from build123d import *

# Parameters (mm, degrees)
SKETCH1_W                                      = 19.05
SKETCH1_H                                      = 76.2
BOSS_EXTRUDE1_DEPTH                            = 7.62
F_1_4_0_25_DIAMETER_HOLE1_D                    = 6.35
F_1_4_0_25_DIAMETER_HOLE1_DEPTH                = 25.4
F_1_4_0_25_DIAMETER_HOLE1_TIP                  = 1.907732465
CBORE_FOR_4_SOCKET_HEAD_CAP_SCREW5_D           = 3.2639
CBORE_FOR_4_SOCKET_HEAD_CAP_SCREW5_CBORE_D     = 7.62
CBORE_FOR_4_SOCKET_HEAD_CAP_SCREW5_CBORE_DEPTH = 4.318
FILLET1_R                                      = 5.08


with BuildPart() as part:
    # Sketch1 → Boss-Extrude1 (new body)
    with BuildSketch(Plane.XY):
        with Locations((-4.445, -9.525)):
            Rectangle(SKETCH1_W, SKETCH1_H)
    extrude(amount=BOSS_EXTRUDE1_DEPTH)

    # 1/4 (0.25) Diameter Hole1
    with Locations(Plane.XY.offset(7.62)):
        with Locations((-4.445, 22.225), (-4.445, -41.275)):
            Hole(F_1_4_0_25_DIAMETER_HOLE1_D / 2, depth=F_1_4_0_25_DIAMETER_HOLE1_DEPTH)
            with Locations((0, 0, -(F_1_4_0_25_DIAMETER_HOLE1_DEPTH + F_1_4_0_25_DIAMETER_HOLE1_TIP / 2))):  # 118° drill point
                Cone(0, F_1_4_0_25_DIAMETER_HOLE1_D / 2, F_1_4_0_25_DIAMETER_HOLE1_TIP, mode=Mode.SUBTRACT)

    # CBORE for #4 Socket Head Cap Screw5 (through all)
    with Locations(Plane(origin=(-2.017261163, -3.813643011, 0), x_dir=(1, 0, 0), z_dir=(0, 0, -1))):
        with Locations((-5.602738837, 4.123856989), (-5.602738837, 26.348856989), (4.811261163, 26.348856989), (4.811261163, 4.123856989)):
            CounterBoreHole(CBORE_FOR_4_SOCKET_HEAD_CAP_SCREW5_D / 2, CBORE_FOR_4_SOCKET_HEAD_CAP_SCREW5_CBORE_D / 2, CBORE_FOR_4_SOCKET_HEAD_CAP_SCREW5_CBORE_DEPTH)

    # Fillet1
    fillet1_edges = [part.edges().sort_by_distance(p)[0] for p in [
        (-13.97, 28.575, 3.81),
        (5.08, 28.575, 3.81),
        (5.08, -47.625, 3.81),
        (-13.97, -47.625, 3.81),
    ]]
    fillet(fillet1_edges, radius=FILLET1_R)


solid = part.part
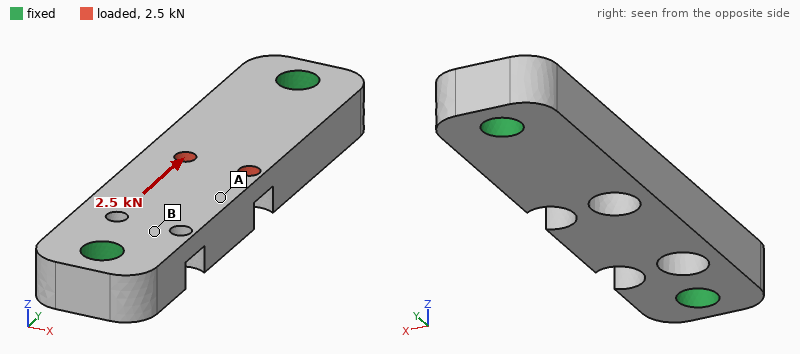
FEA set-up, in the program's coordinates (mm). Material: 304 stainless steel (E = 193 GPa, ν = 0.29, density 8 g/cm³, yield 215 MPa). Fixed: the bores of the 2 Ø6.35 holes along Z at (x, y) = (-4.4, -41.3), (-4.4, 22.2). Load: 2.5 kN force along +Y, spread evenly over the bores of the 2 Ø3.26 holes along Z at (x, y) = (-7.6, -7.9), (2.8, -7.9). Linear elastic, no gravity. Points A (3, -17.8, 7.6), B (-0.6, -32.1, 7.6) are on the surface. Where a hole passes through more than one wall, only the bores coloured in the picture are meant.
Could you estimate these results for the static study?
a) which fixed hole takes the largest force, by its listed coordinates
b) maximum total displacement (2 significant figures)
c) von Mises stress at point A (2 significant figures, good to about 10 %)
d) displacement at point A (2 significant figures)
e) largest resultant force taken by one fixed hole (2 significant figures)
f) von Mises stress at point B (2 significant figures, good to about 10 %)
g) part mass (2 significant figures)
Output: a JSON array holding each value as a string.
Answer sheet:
["(-4.4, 22.2)", "3.5 µm", "22 MPa", "2.2 µm", "1.5 kN", "11 MPa", "77 g"]
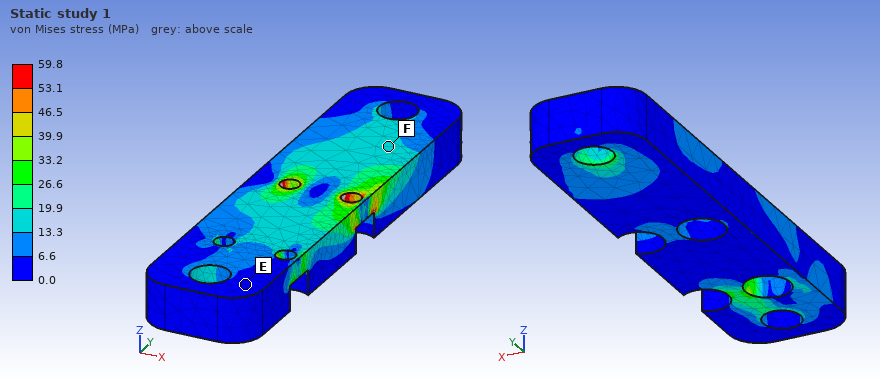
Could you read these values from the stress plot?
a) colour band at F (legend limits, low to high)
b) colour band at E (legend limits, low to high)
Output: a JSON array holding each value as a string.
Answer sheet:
["13.3 to 19.9 MPa", "0.0 to 6.6 MPa"]
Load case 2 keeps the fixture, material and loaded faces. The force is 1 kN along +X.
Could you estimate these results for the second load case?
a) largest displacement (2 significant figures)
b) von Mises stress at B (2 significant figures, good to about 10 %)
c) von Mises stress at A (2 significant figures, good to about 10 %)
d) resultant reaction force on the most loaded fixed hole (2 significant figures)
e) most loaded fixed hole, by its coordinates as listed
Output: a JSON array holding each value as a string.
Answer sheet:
["7.3 µm", "14 MPa", "10 MPa", "560 N", "(-4.4, 22.2)"]
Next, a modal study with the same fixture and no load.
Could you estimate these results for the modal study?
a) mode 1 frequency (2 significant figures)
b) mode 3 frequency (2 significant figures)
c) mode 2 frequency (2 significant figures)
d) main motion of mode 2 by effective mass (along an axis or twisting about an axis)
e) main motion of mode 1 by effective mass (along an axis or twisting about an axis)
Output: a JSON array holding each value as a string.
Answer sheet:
["8800 Hz", "15 kHz", "13 kHz", "along X", "along Z"]
